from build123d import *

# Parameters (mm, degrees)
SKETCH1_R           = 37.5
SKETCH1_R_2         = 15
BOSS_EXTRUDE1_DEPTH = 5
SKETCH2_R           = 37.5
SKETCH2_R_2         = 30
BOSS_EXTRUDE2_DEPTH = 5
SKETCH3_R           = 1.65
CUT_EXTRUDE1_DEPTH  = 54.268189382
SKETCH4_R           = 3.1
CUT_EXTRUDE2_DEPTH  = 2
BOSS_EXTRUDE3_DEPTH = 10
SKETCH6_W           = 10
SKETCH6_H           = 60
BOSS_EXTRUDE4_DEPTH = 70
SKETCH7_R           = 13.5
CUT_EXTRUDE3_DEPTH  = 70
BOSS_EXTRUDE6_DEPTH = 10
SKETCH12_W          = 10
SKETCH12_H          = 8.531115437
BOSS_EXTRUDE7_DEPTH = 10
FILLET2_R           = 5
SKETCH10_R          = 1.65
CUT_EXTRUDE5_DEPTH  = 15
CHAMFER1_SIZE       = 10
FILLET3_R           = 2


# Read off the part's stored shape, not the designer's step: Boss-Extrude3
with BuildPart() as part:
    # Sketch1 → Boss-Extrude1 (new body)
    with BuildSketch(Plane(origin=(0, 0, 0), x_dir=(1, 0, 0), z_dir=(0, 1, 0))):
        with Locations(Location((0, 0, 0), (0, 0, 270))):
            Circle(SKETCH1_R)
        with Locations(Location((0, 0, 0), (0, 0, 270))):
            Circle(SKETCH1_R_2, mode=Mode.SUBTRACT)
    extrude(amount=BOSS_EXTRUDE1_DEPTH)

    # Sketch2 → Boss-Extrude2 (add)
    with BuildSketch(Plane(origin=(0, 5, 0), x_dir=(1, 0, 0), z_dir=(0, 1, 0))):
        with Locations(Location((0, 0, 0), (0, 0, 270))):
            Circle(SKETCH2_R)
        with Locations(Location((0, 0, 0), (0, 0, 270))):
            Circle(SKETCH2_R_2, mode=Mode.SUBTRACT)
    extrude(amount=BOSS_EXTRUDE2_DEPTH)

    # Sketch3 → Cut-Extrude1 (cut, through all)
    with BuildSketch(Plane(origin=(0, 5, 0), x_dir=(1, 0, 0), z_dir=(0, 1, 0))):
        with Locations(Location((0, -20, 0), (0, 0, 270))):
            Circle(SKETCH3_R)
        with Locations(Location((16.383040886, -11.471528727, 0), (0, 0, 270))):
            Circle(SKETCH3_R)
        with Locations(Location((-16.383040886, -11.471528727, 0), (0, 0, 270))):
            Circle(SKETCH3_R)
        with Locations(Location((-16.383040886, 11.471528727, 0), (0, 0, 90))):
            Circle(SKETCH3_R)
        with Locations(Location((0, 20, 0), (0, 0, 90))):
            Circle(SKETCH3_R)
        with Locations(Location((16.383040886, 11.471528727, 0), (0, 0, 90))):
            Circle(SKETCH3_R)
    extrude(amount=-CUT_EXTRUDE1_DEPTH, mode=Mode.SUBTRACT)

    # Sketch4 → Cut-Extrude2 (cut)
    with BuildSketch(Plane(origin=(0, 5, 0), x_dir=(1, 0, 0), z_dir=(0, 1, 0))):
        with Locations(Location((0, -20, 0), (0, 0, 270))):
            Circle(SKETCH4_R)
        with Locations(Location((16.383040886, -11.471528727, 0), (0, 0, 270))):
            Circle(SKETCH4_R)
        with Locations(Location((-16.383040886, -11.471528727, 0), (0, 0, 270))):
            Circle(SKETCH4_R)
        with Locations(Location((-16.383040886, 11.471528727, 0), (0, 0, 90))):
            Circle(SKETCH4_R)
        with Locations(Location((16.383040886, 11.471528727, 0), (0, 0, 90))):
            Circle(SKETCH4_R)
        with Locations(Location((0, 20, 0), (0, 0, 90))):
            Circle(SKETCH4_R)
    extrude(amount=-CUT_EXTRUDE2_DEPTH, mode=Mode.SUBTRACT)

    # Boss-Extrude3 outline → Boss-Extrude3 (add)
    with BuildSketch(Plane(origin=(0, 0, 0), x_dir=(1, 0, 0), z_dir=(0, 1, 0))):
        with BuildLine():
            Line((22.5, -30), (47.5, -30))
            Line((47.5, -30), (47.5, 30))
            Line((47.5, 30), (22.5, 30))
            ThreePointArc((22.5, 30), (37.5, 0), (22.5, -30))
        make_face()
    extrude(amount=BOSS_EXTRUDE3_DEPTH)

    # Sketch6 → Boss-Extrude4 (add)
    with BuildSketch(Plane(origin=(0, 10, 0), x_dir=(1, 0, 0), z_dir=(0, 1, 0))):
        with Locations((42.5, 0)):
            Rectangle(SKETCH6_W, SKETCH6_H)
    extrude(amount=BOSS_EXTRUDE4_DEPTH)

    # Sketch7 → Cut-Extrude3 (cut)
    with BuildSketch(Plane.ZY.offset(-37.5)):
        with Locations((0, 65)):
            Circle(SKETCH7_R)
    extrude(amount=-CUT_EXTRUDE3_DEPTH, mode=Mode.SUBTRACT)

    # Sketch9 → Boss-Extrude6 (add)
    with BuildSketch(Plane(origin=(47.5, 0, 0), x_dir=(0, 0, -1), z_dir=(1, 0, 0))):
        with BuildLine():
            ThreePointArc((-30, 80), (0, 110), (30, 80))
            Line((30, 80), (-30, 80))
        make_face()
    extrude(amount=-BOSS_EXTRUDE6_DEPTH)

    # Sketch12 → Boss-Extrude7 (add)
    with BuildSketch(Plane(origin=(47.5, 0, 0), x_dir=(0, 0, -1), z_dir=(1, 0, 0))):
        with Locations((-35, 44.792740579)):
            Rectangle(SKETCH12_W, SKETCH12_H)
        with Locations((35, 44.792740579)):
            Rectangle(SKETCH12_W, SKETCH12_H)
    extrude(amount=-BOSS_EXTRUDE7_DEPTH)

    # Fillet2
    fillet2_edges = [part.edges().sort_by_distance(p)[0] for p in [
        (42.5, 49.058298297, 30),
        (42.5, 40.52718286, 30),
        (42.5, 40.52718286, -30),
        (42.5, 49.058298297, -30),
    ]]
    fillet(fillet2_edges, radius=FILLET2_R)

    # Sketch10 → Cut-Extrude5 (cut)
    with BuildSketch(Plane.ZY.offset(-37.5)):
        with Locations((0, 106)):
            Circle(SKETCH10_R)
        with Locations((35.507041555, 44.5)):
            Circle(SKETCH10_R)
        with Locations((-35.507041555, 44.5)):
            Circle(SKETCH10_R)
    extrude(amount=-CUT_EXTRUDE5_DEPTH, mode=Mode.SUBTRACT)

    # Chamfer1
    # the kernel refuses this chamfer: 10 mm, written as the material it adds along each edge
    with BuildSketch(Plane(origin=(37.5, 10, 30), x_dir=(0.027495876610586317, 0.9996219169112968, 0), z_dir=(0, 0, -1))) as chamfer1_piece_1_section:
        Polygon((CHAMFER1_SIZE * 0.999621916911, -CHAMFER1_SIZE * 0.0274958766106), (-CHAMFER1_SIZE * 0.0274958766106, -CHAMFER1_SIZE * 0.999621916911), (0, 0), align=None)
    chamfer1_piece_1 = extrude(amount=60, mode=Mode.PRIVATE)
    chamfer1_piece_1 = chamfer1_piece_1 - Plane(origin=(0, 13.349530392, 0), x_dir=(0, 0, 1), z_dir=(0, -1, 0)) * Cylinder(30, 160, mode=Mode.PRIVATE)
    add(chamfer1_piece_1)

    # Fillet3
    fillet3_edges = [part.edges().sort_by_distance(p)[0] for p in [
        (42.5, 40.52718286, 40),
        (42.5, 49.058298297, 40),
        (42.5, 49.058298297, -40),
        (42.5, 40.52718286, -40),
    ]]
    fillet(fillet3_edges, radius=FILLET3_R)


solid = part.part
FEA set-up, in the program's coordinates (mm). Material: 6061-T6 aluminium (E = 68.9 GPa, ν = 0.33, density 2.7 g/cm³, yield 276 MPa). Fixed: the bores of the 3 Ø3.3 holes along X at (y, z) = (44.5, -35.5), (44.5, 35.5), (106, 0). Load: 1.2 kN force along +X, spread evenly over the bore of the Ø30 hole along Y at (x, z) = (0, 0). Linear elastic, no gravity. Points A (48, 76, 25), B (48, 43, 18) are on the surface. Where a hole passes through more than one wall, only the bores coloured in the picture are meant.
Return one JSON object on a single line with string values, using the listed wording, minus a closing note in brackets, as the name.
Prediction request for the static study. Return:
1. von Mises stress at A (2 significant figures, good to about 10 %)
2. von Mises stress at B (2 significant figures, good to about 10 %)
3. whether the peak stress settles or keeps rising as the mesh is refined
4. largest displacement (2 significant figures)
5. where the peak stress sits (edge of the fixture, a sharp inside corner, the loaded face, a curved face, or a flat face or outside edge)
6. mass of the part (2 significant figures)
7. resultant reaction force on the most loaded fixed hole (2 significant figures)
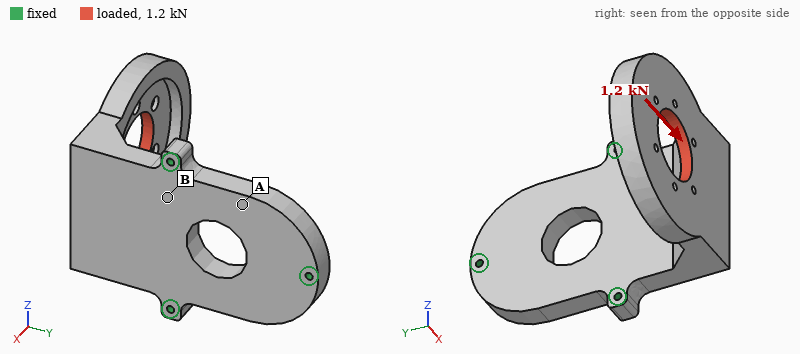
{"von Mises stress at A": "14 MPa", "von Mises stress at B": "39 MPa", "whether the peak stress settles or keeps rising as the mesh is refined": "keeps rising", "largest displacement": "0.47 mm", "where the peak stress sits": "edge of the fixture", "mass of the part": "240 g", "resultant reaction force on the most loaded fixed hole": "860 N"}
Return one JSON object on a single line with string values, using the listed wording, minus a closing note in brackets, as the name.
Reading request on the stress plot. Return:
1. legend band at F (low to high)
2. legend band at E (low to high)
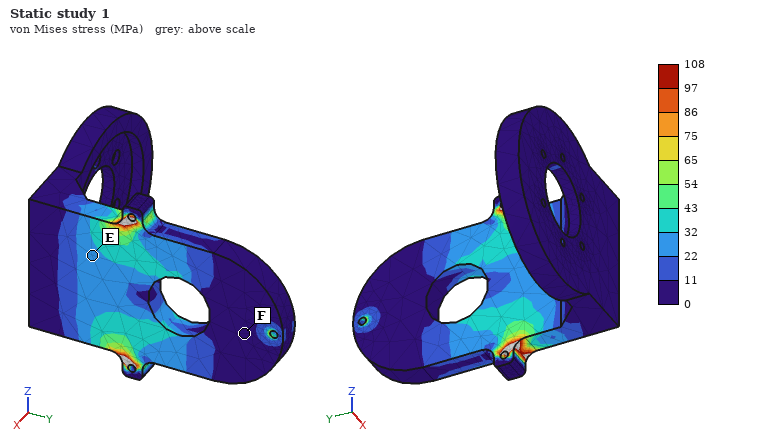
{"legend band at F": "0 to 11 MPa", "legend band at E": "22 to 32 MPa"}
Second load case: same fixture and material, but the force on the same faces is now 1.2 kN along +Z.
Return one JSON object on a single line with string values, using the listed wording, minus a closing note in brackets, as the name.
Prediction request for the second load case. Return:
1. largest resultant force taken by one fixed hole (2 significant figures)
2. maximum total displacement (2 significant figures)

{"largest resultant force taken by one fixed hole": "1.3 kN", "maximum total displacement": "0.19 mm"}
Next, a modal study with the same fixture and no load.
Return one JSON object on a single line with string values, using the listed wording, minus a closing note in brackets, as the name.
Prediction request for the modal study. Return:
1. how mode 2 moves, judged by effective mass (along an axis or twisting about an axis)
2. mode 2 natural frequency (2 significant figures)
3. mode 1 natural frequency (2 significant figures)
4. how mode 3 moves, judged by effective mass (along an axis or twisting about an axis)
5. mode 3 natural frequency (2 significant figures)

{"how mode 2 moves, judged by effective mass": "along Z", "mode 2 natural frequency": "1600 Hz", "mode 1 natural frequency": "760 Hz", "how mode 3 moves, judged by effective mass": "along X", "mode 3 natural frequency": "1900 Hz"}
